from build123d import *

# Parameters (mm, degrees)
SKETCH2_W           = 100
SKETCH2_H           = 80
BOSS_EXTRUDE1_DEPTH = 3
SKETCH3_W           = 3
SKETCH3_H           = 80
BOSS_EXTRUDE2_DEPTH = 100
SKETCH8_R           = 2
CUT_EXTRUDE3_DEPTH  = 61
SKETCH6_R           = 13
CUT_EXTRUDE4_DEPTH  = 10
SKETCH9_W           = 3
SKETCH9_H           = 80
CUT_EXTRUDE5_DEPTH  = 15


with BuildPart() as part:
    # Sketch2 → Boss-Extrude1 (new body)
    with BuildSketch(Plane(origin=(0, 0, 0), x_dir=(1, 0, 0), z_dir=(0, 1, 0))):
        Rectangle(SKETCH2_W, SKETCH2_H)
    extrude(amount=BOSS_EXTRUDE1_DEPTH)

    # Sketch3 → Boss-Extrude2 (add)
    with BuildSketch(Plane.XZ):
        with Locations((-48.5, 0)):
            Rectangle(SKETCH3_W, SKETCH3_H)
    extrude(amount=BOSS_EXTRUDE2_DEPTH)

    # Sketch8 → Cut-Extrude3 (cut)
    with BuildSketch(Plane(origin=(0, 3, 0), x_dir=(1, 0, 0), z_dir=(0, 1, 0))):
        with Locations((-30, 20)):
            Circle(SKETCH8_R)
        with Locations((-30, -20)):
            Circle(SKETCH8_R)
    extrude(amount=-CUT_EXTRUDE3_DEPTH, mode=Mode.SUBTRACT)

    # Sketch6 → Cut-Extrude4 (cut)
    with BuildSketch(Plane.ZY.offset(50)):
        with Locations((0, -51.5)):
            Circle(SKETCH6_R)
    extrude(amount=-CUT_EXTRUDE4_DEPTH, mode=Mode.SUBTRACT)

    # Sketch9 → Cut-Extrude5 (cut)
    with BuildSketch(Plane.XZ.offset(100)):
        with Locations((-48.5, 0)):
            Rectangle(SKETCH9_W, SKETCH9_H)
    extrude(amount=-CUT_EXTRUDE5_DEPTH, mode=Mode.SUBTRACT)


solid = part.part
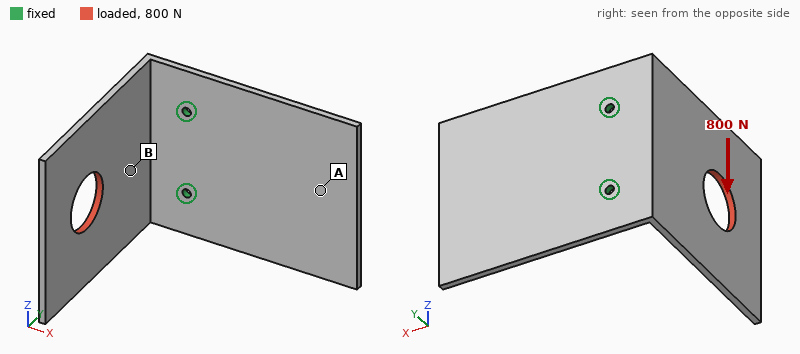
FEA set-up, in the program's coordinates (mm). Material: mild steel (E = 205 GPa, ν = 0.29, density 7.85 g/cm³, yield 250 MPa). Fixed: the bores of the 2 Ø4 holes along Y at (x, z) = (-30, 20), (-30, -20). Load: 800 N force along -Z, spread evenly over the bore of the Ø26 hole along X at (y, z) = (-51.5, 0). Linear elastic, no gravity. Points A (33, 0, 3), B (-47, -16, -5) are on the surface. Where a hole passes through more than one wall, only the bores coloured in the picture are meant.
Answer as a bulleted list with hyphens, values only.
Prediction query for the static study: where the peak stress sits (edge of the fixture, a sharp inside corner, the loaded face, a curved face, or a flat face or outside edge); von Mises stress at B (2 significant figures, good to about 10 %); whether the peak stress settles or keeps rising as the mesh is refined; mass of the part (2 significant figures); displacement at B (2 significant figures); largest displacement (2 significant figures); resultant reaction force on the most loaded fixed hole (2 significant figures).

- edge of the fixture
- 40 MPa
- keeps rising
- 340 g
- 0.069 mm
- 0.37 mm
- 1.1 kN
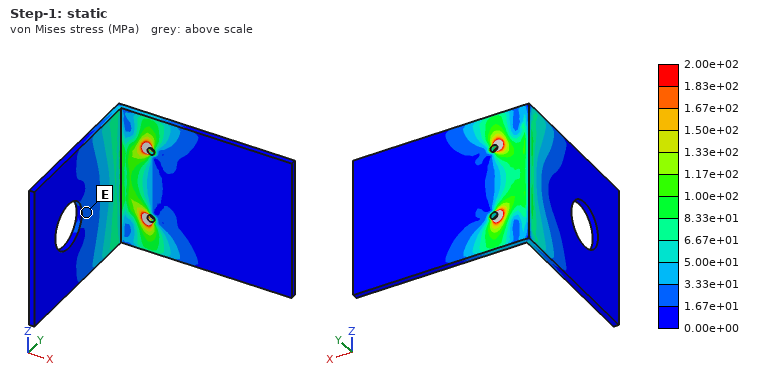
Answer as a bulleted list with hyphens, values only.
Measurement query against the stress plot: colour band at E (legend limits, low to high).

- 1.67e+01 to 3.33e+01 MPa
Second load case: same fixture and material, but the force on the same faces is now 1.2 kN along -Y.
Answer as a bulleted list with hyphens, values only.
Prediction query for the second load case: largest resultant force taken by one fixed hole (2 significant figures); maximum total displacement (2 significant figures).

- 600 N
- 0.60 mm
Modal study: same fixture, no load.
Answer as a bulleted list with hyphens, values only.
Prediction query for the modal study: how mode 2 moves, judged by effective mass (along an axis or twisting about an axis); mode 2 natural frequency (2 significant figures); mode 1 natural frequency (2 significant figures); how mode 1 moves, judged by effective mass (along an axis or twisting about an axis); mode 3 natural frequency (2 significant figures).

- along Y
- 380 Hz
- 250 Hz
- along X
- 680 Hz
